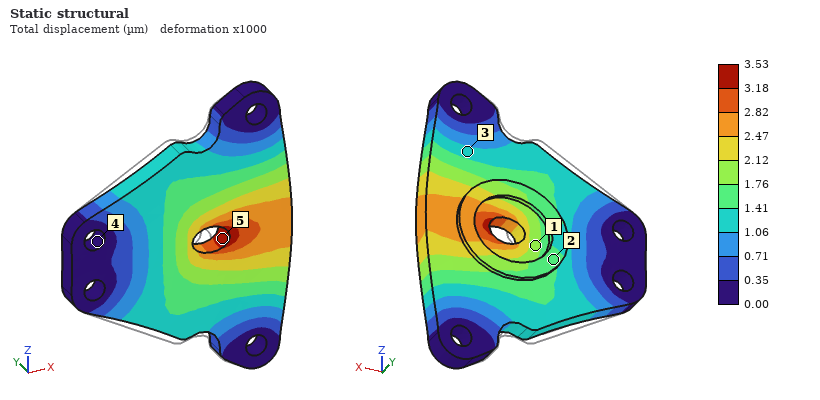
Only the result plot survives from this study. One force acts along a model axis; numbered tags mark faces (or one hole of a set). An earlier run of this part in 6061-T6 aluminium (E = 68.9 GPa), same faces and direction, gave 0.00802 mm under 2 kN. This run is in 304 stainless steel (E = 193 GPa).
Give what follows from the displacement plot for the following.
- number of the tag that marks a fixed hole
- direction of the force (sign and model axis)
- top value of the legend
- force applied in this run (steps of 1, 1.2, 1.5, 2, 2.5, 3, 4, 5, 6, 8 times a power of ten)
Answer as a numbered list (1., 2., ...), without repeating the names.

1. 4
2. +X
3. 3.53 µm
4. 2.5 kN
